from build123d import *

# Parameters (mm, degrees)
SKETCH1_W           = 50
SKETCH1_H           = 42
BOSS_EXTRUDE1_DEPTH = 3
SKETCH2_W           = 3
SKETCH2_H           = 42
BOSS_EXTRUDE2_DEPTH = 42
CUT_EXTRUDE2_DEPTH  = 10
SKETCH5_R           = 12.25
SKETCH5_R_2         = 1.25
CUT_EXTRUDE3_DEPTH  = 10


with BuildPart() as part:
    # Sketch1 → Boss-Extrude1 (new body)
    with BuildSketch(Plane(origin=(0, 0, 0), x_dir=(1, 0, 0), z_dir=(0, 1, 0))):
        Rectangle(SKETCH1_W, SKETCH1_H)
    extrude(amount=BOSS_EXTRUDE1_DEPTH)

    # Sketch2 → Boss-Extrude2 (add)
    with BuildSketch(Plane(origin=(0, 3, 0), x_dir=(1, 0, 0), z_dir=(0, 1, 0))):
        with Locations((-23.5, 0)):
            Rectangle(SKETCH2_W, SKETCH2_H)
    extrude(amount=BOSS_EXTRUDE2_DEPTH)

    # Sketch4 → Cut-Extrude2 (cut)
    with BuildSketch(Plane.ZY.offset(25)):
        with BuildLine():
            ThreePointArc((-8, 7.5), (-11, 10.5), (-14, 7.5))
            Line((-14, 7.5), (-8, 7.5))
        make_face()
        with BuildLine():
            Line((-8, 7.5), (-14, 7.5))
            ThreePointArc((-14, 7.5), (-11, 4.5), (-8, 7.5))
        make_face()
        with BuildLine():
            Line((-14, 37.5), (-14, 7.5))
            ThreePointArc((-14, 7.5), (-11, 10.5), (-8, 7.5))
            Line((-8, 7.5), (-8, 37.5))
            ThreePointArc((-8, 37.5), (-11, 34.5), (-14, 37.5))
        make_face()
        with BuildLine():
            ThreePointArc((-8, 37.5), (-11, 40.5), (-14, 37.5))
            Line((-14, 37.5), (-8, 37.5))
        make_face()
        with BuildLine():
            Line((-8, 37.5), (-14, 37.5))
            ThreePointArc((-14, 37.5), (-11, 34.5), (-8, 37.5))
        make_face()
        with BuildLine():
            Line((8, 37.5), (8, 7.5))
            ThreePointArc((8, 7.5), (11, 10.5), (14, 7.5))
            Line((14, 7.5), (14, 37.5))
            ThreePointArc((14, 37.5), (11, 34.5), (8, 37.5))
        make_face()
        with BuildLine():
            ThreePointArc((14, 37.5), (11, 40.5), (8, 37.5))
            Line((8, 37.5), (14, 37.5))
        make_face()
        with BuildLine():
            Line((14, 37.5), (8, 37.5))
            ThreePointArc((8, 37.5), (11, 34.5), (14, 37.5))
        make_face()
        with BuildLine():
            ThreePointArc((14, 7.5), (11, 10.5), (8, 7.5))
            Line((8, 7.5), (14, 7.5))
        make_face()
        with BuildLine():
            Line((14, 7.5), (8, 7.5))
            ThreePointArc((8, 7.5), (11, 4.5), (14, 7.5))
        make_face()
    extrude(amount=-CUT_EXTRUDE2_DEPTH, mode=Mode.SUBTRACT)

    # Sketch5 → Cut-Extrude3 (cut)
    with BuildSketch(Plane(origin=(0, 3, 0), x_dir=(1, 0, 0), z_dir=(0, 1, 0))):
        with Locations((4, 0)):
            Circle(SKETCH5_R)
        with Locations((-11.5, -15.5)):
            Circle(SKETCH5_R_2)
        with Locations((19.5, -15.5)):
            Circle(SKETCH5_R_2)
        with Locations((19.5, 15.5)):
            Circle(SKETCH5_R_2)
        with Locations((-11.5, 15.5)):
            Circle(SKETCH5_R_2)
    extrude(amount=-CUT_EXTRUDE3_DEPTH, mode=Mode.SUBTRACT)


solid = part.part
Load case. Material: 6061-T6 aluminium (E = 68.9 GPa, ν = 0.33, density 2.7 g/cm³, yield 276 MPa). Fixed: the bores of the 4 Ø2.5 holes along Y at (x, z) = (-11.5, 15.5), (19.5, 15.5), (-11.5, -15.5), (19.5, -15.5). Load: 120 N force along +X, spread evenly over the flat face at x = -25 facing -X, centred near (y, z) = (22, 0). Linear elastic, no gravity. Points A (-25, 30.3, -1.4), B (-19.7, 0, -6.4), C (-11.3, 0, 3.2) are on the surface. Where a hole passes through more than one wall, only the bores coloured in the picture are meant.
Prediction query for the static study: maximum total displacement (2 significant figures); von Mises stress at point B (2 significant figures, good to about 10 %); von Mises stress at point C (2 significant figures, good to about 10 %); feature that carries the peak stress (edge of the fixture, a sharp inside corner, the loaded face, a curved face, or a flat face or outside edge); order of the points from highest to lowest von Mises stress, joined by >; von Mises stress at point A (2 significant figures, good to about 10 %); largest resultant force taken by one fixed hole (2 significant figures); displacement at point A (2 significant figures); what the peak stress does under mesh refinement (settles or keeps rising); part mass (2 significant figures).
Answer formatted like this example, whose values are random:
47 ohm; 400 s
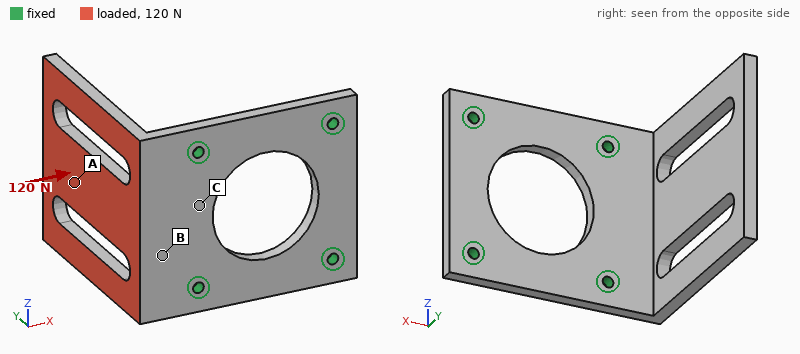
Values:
0.45 mm; 33 MPa; 16 MPa; edge of the fixture; B > C > A; 7.3 MPa; 61 N; 0.27 mm; keeps rising; 24 g
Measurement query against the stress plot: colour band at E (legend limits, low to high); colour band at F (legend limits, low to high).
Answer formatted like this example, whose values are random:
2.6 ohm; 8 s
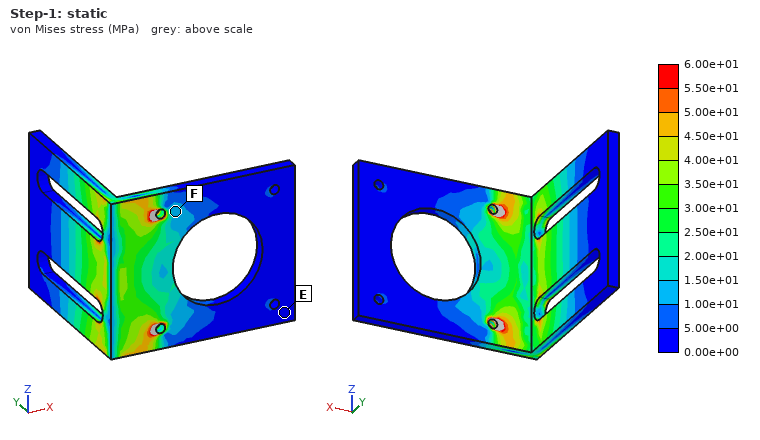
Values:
0.00e+00 to 5.00e+00 MPa; 1.00e+01 to 1.50e+01 MPa
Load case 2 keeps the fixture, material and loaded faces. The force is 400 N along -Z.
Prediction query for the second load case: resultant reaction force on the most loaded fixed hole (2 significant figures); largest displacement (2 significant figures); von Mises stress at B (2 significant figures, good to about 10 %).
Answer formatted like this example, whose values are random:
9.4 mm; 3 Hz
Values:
370 N; 0.15 mm; 27 MPa
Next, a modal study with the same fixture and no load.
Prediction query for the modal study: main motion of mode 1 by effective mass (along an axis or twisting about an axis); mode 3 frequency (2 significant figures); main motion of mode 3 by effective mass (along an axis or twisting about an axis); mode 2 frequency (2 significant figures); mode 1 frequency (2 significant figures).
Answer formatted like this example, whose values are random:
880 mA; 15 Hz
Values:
along X; 3200 Hz; along Z; 2400 Hz; 910 Hz
